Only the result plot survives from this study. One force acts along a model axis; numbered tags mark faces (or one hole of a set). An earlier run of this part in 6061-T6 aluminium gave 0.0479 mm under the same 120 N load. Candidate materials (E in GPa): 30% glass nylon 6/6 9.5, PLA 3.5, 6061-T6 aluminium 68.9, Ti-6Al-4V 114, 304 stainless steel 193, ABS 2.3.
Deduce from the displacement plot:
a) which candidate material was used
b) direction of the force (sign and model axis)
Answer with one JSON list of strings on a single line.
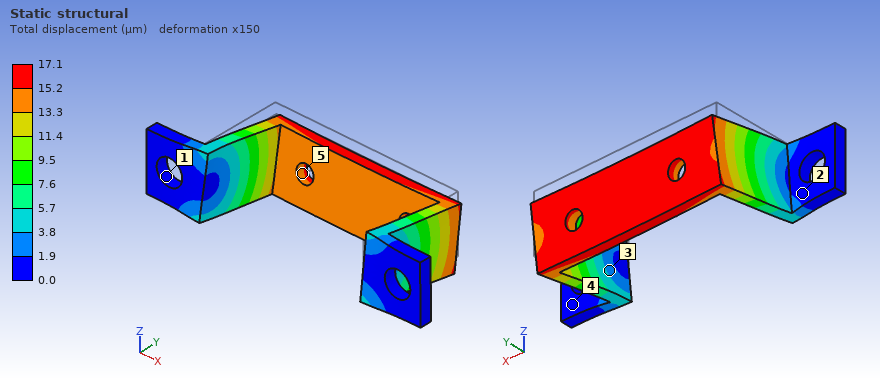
["304 stainless steel", "-Z"]
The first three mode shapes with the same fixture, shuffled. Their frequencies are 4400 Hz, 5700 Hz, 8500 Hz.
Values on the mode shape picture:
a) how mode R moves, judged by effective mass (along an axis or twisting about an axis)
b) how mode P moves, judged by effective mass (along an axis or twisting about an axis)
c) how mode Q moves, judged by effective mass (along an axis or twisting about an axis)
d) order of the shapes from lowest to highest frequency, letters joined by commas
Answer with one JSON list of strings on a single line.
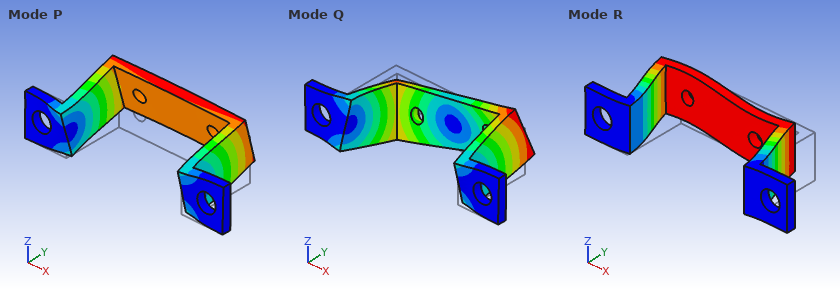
["along X", "along Z", "twisting about Y", "R, P, Q"]
